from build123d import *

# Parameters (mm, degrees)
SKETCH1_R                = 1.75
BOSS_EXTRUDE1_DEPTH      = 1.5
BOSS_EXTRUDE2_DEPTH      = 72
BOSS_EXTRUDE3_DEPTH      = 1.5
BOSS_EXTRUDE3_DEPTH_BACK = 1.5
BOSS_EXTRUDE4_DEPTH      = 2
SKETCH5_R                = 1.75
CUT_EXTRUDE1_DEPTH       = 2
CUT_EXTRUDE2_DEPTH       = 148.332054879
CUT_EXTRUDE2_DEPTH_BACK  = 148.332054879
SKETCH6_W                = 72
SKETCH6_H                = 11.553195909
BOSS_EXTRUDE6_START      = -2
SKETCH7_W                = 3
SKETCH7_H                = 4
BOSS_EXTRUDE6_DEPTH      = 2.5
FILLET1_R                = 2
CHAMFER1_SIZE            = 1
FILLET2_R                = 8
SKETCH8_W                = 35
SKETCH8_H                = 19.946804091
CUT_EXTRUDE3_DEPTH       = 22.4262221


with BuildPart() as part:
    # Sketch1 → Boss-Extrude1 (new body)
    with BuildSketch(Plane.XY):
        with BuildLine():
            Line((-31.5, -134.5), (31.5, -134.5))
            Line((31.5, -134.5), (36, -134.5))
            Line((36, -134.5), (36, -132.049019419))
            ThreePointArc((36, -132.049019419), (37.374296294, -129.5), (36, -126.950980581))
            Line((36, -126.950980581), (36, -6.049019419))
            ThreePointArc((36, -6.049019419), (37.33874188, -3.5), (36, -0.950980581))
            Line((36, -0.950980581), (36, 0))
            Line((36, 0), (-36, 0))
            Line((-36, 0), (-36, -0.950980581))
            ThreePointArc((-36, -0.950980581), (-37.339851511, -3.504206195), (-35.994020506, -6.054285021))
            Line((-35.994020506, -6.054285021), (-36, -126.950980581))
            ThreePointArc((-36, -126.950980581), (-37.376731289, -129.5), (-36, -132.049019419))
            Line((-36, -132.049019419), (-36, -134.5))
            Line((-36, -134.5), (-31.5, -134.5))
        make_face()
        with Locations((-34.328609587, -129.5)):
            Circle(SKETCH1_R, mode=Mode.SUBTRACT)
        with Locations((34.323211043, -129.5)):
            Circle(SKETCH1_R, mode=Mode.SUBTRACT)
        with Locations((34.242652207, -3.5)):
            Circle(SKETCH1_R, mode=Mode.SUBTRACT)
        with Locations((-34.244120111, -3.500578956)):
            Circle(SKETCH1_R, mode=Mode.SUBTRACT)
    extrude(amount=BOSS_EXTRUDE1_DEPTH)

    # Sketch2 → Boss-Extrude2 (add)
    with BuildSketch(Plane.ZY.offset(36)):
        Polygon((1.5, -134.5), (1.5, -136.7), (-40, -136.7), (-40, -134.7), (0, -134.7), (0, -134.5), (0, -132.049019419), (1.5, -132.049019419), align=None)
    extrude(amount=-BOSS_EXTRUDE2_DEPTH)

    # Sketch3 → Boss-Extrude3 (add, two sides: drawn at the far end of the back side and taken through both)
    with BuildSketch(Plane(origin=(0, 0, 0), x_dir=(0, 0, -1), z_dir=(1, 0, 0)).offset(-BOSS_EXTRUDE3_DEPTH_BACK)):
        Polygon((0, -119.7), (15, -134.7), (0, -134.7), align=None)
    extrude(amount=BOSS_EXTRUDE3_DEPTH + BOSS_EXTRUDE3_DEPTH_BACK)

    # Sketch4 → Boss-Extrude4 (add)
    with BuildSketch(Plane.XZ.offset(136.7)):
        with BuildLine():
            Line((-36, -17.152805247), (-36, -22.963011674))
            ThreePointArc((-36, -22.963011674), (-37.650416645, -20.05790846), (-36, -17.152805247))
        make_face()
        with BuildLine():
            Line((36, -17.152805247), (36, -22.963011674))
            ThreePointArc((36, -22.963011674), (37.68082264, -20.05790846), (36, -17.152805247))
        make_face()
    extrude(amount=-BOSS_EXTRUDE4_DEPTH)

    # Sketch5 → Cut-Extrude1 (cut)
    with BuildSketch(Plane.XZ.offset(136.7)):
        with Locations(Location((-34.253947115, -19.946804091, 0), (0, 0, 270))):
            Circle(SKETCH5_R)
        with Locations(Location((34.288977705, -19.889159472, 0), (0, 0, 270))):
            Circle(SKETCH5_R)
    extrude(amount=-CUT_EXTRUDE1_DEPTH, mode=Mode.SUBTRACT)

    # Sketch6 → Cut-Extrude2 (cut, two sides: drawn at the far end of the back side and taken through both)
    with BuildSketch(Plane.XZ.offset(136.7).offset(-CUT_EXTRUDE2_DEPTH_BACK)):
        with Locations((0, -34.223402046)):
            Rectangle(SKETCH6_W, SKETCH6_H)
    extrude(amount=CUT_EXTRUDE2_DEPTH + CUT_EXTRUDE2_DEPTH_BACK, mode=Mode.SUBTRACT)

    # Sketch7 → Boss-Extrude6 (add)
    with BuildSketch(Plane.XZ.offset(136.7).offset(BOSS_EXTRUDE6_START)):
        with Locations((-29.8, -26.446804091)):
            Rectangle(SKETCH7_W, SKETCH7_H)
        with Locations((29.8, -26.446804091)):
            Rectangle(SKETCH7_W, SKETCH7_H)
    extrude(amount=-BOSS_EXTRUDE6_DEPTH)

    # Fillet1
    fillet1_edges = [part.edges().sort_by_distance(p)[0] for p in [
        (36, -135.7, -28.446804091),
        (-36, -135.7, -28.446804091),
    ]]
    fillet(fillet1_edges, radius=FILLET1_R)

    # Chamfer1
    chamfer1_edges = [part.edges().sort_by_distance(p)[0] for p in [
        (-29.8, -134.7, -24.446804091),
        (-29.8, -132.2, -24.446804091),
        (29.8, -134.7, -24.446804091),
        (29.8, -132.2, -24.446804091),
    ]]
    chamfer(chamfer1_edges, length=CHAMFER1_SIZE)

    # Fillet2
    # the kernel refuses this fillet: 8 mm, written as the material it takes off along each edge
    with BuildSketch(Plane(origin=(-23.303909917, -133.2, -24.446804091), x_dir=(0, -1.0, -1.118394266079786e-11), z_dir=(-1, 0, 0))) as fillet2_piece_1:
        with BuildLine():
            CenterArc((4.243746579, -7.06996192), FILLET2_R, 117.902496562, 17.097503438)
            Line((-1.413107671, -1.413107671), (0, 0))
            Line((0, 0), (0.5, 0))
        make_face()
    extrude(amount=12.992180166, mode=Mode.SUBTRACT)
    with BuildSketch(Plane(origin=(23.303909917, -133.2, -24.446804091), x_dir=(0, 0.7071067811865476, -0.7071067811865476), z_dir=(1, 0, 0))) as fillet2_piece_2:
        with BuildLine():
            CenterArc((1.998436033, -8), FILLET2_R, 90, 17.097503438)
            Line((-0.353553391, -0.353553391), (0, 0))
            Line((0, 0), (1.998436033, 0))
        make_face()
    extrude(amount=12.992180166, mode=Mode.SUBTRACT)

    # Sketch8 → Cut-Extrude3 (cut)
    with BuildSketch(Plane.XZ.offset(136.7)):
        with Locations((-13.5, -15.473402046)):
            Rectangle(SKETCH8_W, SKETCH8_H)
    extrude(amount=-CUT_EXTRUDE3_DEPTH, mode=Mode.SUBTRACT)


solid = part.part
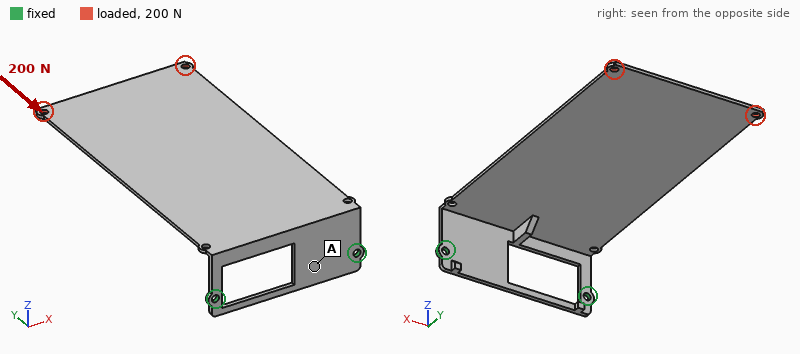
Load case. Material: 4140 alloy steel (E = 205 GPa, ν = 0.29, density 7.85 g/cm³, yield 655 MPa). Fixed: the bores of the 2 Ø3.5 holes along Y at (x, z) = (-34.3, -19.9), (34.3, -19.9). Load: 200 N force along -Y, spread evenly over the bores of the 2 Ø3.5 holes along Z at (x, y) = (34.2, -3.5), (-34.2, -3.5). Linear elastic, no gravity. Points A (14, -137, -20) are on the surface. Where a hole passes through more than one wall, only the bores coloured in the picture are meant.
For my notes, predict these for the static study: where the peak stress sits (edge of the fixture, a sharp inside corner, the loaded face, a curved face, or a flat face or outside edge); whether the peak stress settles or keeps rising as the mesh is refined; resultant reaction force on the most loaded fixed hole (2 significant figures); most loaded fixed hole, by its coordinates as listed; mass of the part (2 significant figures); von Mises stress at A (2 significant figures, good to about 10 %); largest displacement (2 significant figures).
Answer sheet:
edge of the fixture
keeps rising
110 N
(34.3, -19.9)
140 g
41 MPa
1.6 mm
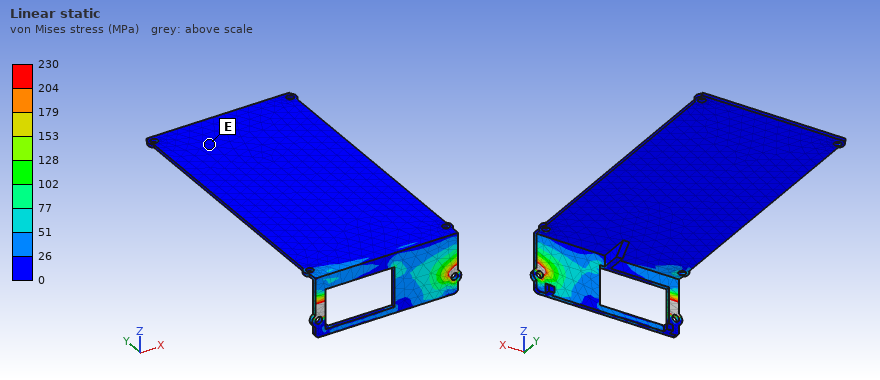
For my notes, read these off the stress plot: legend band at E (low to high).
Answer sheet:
0 to 26 MPa
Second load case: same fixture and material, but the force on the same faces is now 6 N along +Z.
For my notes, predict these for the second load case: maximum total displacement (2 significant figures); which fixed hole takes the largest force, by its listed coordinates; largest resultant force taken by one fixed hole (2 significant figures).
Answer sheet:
1.6 mm
(34.3, -19.9)
5.1 N
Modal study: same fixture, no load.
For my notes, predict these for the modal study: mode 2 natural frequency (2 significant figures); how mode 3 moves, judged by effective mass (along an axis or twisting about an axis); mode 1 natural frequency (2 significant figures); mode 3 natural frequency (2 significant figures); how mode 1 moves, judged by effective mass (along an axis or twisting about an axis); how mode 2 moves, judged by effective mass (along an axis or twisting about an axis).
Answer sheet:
240 Hz
along X
56 Hz
300 Hz
along Z
along X
